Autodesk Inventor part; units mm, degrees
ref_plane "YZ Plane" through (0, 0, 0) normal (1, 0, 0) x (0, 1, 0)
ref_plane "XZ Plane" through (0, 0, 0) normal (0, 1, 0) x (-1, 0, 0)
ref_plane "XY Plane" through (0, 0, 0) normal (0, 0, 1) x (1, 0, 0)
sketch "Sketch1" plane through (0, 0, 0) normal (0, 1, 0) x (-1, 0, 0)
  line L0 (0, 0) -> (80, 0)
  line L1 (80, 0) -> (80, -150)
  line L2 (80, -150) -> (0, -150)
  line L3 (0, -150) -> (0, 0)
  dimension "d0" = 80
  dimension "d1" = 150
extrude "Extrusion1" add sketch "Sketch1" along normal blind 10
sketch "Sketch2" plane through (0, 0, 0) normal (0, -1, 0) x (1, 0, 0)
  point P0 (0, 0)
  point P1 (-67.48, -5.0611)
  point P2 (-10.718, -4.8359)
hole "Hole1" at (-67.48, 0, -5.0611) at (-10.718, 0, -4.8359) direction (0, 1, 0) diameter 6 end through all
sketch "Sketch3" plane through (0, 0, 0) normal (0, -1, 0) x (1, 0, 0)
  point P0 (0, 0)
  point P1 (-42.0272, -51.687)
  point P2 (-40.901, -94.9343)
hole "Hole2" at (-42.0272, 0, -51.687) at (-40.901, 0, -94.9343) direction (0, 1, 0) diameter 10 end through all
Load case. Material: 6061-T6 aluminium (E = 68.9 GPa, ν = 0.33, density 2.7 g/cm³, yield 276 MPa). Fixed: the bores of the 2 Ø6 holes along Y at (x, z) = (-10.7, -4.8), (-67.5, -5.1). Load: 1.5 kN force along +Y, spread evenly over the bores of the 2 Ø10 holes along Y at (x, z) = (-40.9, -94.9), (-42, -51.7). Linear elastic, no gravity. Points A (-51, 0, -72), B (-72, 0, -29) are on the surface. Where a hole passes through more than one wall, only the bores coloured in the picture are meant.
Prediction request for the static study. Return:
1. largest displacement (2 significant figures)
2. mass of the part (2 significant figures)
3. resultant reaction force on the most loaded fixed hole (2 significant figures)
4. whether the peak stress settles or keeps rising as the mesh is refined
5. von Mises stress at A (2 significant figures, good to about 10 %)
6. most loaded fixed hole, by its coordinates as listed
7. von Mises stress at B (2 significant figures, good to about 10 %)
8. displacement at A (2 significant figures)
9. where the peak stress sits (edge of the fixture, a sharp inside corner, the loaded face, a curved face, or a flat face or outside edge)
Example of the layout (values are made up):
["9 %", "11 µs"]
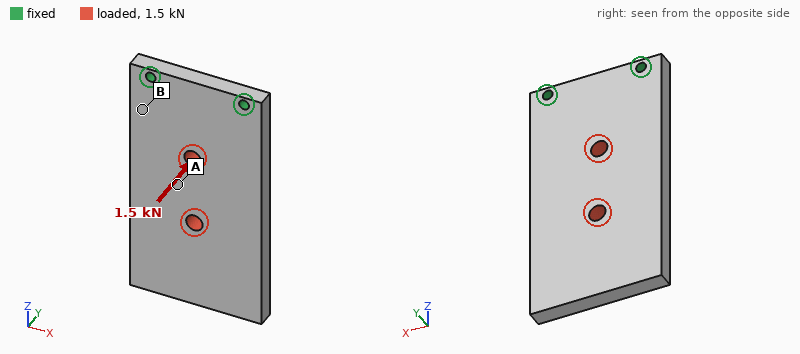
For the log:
["1.3 mm", "320 g", "830 N", "keeps rising", "17 MPa", "(-67.5, -5.1)", "56 MPa", "0.47 mm", "edge of the fixture"]
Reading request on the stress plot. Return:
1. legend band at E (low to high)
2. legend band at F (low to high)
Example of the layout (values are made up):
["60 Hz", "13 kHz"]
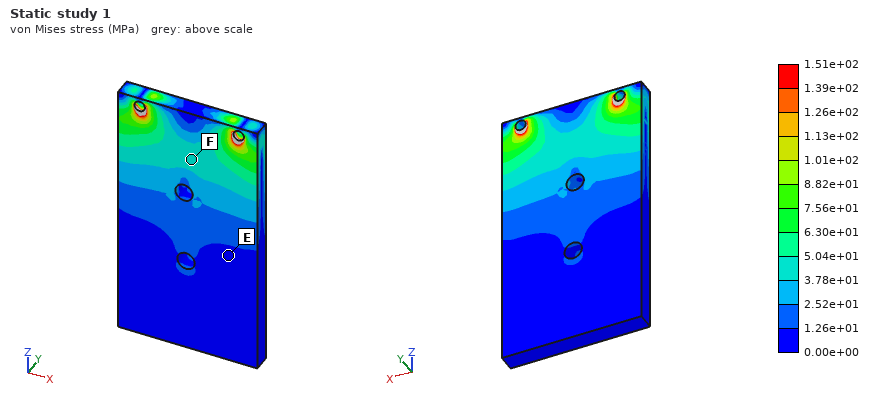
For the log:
["0.00e+00 to 1.26e+01 MPa", "3.78e+01 to 5.04e+01 MPa"]
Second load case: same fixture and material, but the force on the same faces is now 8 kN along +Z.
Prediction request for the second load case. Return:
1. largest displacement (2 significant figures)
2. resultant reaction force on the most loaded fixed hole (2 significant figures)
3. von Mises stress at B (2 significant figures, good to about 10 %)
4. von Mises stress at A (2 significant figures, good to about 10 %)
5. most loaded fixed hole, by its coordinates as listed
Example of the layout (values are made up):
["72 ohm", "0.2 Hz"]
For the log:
["16 µm", "4.4 kN", "12 MPa", "7.2 MPa", "(-67.5, -5.1)"]
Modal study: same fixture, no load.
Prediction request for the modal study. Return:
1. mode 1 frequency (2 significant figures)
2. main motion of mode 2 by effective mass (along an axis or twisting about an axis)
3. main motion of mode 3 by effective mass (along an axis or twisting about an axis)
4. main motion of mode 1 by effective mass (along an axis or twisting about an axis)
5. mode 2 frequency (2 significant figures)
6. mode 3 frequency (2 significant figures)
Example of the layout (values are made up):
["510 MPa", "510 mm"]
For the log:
["350 Hz", "twisting about Z", "along Y", "along Y", "1400 Hz", "2200 Hz"]
